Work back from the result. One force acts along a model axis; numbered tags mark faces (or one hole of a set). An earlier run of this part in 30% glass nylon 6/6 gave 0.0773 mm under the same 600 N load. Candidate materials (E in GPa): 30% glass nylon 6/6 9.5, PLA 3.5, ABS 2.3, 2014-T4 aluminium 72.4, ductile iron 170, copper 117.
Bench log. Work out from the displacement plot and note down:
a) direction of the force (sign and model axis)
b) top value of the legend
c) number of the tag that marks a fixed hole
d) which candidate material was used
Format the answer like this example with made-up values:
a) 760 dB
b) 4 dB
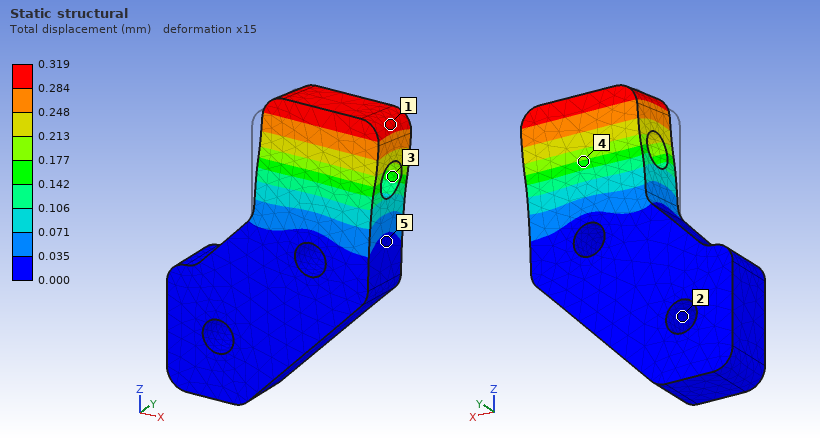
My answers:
a) +Y
b) 0.319 mm
c) 2
d) ABS
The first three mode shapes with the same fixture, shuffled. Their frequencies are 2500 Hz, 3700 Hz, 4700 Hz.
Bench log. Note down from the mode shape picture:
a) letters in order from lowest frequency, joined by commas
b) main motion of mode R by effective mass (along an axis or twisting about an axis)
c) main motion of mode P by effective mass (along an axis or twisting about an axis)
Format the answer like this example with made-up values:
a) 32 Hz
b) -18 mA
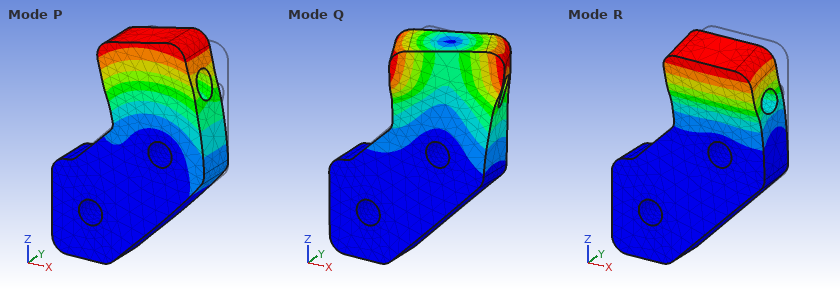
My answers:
a) R, P, Q
b) along Y
c) along X
